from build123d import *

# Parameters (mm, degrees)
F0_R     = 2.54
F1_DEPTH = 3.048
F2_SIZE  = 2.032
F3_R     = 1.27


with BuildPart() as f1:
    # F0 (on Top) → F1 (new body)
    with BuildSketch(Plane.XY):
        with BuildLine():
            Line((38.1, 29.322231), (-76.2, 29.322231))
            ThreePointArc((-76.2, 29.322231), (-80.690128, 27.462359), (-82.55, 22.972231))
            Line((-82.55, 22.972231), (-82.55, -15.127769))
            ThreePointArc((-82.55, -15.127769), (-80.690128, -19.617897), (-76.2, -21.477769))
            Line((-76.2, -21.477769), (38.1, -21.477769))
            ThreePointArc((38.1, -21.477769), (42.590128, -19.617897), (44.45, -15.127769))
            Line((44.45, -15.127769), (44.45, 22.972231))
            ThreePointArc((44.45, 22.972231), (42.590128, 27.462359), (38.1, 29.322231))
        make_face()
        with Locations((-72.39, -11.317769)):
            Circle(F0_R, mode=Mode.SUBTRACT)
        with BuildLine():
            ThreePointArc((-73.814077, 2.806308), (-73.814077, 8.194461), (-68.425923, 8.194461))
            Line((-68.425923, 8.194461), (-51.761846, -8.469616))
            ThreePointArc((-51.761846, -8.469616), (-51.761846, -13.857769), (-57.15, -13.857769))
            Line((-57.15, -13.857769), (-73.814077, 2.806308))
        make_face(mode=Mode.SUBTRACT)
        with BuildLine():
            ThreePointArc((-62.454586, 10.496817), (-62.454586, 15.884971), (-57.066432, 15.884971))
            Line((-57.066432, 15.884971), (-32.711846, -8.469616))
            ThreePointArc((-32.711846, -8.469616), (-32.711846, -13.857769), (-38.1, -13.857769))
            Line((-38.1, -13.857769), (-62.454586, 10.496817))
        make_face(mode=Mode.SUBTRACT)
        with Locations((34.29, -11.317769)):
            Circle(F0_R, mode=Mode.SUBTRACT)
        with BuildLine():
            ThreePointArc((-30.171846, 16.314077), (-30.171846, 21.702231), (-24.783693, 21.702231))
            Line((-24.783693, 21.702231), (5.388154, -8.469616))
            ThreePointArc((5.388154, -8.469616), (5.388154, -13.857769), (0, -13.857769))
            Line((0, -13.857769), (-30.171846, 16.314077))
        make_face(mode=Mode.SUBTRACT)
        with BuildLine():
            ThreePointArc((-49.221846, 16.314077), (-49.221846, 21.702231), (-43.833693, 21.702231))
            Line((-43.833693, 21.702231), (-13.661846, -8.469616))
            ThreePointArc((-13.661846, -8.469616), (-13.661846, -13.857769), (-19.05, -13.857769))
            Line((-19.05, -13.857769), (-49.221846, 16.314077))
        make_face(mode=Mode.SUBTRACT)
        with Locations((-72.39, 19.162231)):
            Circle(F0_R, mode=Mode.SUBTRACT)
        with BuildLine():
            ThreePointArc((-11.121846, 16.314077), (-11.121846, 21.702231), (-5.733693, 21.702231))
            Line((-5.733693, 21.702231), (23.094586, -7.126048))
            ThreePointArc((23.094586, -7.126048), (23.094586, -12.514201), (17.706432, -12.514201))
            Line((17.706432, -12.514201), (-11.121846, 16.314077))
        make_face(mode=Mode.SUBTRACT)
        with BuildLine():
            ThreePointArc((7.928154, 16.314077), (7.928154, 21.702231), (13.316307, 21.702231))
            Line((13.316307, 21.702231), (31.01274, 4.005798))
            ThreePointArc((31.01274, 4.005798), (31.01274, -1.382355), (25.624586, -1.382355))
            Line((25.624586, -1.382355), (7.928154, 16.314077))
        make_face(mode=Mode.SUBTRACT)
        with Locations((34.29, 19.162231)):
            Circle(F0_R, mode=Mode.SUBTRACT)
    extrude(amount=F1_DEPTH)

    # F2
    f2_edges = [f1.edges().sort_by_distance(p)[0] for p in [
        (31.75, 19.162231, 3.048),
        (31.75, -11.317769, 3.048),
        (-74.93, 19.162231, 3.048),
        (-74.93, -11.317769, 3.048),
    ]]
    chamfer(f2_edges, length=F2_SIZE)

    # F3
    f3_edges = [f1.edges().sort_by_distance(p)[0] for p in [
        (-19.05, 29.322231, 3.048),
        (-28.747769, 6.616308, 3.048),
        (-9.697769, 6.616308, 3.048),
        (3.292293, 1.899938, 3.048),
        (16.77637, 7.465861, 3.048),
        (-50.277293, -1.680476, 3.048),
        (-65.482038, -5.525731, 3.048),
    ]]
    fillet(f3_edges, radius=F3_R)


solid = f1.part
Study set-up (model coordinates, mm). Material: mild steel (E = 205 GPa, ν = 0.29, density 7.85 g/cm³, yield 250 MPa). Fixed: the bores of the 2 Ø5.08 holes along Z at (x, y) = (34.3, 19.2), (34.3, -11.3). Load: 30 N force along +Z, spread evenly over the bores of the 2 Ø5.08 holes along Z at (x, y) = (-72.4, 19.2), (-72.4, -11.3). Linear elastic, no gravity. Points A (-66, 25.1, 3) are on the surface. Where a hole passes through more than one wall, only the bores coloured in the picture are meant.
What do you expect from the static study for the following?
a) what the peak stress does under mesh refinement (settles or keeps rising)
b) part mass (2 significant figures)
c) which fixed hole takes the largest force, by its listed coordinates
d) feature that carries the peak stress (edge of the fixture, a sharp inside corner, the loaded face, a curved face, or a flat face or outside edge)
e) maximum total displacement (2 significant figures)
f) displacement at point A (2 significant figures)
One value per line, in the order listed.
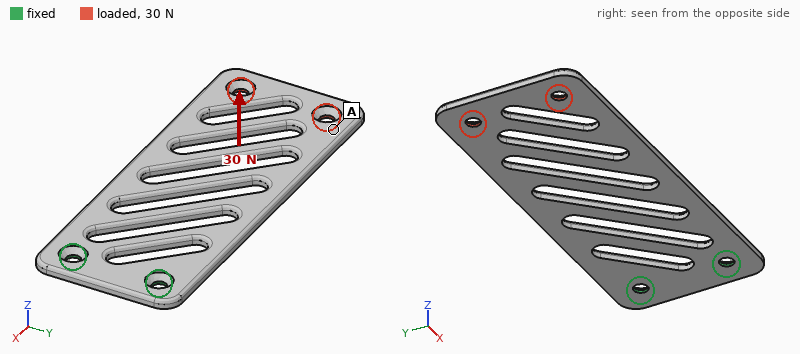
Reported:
keeps rising
100 g
(34.3, 19.2)
edge of the fixture
1.4 mm
1.0 mm
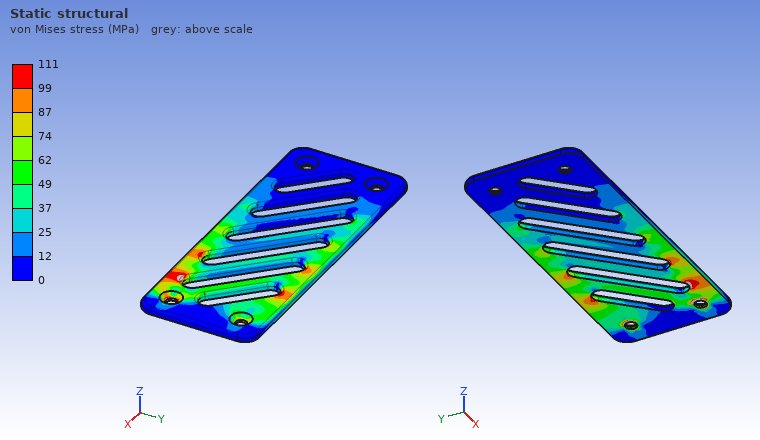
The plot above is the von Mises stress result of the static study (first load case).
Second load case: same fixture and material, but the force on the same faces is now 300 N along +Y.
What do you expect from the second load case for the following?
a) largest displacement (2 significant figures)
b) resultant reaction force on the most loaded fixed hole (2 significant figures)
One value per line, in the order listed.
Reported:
0.13 mm
980 N
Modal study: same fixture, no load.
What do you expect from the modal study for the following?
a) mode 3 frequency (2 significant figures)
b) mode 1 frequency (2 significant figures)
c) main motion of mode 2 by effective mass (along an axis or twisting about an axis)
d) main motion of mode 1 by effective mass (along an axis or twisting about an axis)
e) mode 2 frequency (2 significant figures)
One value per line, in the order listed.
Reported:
910 Hz
140 Hz
twisting about X
along Z
630 Hz
